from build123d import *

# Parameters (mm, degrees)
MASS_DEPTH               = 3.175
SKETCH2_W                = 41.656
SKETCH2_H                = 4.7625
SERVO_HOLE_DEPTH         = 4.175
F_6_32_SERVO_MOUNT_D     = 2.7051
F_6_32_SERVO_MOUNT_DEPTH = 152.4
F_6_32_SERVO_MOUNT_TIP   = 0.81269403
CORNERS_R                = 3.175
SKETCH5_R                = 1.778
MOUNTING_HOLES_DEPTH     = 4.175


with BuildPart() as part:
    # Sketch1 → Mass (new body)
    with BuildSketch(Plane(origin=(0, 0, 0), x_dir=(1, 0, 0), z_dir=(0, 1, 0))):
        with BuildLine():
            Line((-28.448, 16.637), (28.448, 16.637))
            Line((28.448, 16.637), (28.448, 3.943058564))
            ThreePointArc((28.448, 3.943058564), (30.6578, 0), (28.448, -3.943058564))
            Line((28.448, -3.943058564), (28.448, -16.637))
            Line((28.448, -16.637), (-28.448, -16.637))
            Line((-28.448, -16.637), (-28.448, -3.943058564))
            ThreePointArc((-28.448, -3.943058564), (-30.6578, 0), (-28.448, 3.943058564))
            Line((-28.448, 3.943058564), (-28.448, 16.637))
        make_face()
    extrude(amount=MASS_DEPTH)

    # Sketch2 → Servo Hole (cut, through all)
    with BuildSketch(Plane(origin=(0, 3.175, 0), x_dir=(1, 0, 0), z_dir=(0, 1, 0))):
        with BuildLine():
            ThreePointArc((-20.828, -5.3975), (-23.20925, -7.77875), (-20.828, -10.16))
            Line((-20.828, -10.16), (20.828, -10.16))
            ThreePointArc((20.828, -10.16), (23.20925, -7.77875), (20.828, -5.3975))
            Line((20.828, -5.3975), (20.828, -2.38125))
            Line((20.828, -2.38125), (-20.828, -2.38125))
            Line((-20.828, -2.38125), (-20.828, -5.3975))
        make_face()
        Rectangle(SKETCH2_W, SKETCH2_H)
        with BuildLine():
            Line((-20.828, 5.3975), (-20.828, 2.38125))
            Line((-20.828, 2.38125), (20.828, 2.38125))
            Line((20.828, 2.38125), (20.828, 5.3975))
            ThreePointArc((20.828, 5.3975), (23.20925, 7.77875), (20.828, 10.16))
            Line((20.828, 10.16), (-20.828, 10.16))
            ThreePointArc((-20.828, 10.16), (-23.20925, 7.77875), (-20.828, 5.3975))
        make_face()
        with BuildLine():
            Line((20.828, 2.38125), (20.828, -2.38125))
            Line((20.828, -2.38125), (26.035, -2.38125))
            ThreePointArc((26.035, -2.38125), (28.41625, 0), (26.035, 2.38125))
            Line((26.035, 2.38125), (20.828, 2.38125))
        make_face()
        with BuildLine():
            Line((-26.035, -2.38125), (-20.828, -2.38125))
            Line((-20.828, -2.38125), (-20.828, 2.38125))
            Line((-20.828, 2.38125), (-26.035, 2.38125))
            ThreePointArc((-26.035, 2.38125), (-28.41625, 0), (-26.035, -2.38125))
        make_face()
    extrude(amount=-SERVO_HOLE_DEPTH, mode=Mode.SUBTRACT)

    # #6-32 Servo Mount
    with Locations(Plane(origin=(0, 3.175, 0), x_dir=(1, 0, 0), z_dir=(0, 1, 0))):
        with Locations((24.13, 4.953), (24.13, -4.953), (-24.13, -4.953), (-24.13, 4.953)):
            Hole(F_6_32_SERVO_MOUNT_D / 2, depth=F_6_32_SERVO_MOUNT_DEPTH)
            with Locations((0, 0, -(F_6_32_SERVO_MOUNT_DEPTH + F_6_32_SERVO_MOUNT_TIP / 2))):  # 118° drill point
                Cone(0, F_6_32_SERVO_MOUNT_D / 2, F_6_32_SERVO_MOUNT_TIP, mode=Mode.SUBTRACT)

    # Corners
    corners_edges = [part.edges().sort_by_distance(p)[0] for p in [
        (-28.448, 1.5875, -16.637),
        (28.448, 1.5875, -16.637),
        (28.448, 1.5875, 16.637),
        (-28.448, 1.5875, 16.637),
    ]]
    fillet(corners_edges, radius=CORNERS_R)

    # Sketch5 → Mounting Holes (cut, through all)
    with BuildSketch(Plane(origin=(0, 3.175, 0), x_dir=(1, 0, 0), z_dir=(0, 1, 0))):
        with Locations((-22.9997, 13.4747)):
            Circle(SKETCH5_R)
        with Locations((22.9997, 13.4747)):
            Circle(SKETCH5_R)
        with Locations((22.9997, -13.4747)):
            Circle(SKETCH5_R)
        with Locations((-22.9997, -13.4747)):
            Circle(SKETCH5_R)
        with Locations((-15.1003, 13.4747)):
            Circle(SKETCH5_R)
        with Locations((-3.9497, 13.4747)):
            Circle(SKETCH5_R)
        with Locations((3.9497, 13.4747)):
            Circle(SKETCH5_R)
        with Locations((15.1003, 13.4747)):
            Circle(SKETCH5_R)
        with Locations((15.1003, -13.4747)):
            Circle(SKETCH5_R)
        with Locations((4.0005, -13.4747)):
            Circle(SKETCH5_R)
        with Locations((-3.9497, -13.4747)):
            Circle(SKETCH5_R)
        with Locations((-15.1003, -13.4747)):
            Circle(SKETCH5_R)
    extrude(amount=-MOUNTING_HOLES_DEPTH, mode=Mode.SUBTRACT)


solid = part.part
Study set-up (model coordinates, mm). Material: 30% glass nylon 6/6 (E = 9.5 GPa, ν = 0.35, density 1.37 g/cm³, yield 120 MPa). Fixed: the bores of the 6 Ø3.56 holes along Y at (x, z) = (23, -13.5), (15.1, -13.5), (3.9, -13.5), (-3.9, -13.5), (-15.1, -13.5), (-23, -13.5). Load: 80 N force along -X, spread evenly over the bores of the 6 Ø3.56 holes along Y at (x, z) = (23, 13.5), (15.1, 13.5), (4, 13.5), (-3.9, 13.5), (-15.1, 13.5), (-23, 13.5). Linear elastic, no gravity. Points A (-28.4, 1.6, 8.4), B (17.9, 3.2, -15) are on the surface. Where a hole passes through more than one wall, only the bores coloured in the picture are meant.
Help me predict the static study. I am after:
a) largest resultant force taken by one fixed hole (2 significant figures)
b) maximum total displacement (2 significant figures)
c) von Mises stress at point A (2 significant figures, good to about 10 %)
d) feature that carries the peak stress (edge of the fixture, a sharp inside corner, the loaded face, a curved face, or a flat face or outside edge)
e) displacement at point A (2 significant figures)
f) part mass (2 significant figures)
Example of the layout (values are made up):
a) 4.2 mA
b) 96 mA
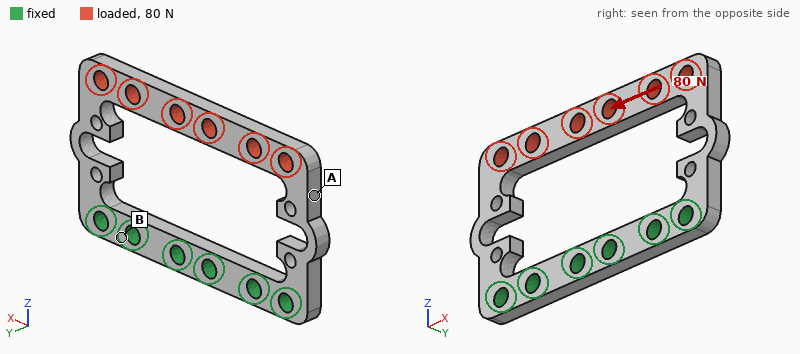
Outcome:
a) 42 N
b) 0.35 mm
c) 20 MPa
d) a curved face
e) 0.29 mm
f) 3.6 g
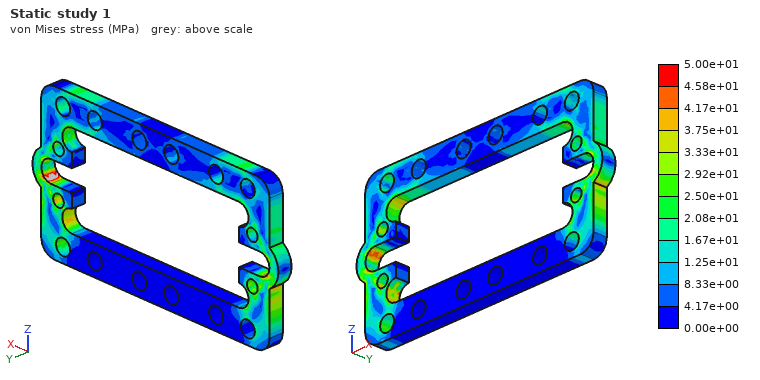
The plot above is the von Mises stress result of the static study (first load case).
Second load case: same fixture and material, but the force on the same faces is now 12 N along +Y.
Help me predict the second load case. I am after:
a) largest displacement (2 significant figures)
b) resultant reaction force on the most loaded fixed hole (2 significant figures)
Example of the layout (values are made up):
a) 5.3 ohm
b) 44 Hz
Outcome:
a) 0.73 mm
b) 7.4 N
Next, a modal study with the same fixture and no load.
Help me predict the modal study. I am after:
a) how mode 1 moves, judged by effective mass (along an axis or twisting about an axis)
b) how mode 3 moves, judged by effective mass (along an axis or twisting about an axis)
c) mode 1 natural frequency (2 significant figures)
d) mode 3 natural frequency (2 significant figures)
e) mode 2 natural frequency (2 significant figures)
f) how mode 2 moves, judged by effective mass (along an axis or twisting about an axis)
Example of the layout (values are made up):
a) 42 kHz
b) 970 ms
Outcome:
a) along Y
b) along X
c) 610 Hz
d) 1900 Hz
e) 1500 Hz
f) twisting about Z
